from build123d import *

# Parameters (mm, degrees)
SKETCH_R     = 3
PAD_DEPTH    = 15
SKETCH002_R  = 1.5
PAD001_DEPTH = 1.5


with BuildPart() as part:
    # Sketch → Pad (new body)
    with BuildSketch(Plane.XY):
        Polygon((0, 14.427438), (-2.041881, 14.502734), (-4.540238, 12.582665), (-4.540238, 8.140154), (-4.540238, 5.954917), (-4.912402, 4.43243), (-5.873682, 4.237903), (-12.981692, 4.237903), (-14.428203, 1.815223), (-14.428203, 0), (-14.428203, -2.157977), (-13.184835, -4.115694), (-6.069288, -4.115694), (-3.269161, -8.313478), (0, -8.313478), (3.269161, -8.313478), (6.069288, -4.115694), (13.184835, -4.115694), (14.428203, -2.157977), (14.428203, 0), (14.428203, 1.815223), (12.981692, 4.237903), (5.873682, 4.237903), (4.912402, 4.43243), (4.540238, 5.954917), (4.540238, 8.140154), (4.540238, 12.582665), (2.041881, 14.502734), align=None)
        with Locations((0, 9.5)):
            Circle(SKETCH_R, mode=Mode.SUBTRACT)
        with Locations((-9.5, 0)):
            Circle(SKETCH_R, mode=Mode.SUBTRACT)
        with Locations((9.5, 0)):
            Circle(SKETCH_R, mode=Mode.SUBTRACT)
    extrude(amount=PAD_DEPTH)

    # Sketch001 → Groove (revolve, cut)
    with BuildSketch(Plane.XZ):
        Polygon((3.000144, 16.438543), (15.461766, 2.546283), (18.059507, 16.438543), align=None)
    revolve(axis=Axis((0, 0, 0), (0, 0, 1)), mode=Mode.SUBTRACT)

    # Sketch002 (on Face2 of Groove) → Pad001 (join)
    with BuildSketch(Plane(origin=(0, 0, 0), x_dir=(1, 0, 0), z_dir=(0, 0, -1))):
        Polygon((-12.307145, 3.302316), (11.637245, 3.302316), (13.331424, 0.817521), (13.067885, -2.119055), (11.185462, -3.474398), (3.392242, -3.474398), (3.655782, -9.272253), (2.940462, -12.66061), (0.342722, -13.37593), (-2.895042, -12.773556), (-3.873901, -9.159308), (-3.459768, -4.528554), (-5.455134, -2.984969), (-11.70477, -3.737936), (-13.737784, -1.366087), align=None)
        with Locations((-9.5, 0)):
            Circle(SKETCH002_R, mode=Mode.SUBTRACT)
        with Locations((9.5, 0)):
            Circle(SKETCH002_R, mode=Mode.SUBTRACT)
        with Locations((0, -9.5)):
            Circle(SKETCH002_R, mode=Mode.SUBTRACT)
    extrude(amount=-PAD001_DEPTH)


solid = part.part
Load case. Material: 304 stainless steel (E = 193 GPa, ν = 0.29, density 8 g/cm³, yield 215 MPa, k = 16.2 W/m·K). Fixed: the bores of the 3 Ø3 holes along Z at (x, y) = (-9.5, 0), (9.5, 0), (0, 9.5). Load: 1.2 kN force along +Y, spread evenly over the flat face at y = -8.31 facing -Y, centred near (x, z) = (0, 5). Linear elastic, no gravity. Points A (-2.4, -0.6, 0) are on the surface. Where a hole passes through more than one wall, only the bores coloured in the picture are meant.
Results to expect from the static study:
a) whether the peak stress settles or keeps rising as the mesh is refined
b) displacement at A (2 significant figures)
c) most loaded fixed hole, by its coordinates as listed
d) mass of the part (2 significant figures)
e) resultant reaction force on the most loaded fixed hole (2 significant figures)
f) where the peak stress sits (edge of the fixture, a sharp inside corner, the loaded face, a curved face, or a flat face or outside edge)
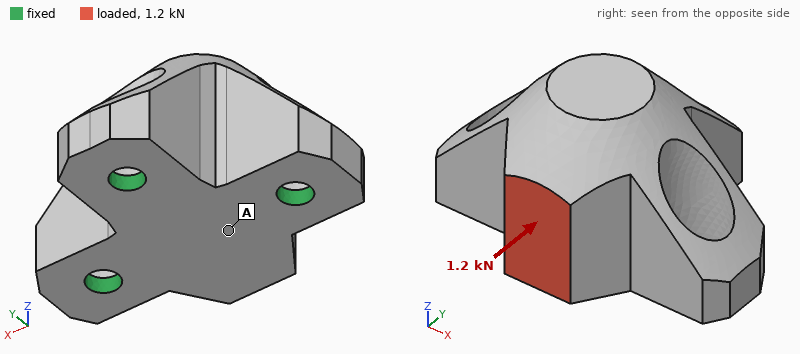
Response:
keeps rising
1.5 µm
(0, 9.5)
26 g
810 N
edge of the fixture
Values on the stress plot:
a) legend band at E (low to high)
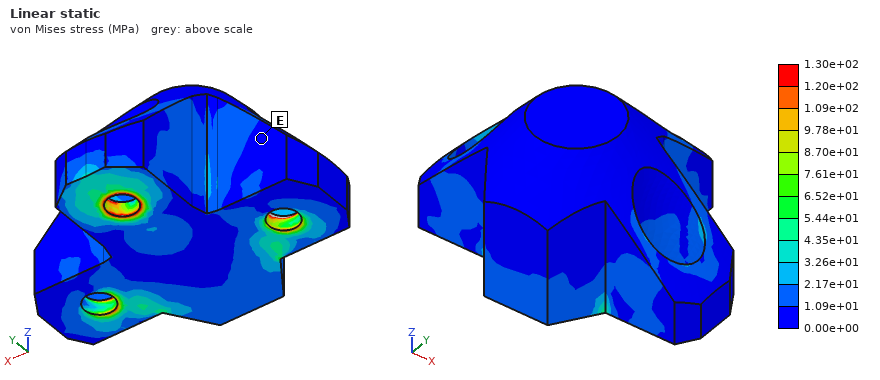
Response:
0.00e+00 to 1.09e+01 MPa
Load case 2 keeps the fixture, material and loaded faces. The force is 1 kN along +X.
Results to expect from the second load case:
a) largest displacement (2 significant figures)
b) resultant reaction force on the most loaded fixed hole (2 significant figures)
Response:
3.9 µm
700 N
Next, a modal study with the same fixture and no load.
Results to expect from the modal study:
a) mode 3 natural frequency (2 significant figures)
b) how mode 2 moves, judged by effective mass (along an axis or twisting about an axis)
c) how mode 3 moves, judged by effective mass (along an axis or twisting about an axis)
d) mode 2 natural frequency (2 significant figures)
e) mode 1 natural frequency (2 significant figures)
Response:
31 kHz
along X
along Z
24 kHz
15 kHz
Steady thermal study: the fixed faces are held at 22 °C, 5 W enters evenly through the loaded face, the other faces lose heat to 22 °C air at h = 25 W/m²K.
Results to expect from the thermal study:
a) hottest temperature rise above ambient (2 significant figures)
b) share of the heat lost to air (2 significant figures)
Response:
42 K
13 %
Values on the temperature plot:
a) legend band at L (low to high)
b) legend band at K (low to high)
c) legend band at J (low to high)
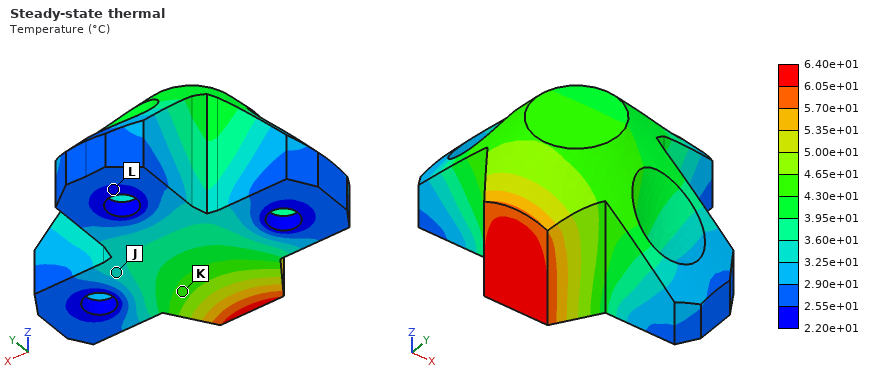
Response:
2.20e+01 to 2.55e+01 °C
4.30e+01 to 4.65e+01 °C
3.25e+01 to 3.60e+01 °C
